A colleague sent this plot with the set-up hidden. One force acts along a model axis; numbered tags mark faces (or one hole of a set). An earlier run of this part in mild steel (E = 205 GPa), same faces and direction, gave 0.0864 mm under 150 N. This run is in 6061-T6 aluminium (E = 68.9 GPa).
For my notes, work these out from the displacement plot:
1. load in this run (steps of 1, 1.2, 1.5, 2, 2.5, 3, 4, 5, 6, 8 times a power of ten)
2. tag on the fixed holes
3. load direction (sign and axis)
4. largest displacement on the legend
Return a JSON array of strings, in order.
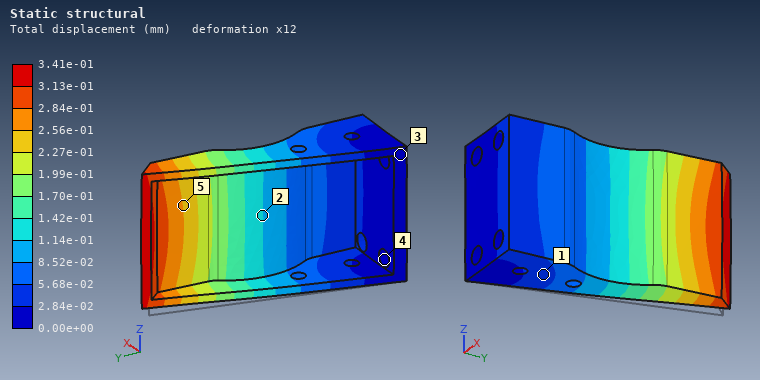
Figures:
["200 N", "4", "+X", "3.41e-01 mm"]
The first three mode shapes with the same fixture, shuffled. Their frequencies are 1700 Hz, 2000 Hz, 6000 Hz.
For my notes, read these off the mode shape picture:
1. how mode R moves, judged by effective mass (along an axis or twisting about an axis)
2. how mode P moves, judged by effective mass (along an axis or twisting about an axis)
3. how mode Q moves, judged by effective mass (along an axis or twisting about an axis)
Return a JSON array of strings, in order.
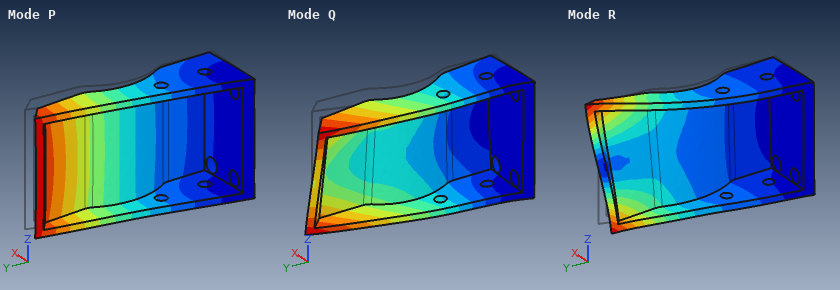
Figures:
["along Z", "along X", "along Z"]
